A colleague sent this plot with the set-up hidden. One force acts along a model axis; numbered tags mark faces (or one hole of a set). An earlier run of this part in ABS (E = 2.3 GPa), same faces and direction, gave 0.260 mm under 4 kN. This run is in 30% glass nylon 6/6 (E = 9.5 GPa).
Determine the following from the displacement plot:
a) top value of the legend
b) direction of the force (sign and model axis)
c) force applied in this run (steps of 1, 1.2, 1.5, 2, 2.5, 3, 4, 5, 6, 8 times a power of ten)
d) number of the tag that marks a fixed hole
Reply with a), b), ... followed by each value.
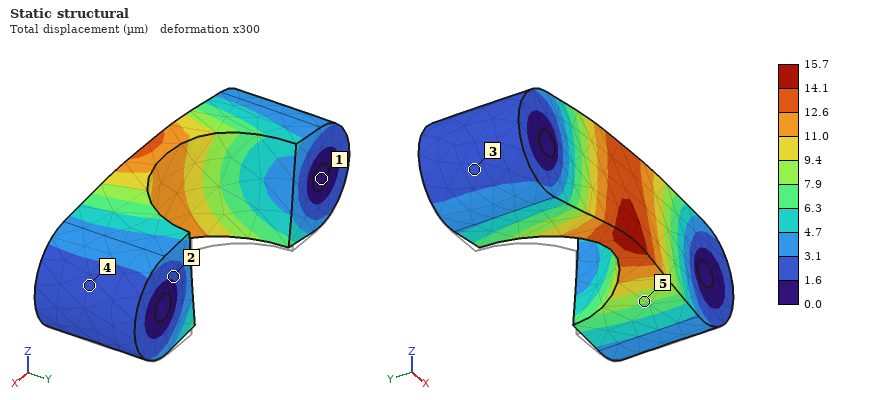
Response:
a) 15.7 µm
b) +Z
c) 1 kN
d) 1
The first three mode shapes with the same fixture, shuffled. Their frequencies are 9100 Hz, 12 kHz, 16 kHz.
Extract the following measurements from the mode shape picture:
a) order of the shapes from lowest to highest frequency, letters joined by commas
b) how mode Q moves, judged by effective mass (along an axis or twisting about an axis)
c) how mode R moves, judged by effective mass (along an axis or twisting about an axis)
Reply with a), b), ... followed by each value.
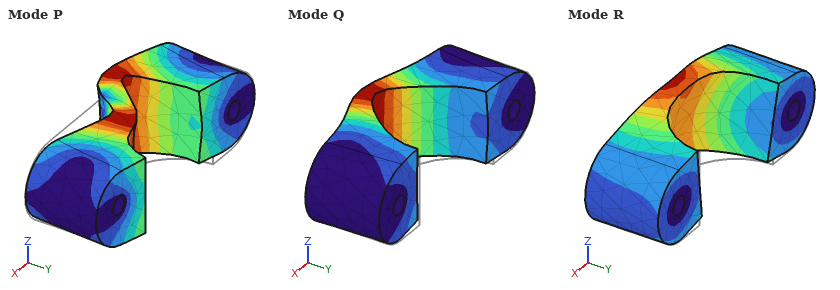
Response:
a) R, Q, P
b) along Y
c) along Z
